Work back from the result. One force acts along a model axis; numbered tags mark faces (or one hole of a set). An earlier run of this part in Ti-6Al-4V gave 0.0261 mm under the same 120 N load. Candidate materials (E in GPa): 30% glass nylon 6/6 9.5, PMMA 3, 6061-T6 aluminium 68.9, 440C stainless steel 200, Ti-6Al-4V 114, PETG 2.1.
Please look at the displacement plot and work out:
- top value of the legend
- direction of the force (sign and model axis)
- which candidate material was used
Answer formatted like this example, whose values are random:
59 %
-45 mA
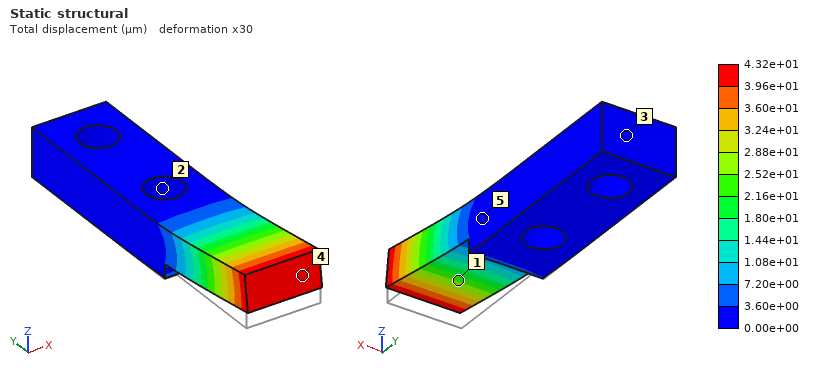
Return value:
4.32e+01 µm
+Z
6061-T6 aluminium
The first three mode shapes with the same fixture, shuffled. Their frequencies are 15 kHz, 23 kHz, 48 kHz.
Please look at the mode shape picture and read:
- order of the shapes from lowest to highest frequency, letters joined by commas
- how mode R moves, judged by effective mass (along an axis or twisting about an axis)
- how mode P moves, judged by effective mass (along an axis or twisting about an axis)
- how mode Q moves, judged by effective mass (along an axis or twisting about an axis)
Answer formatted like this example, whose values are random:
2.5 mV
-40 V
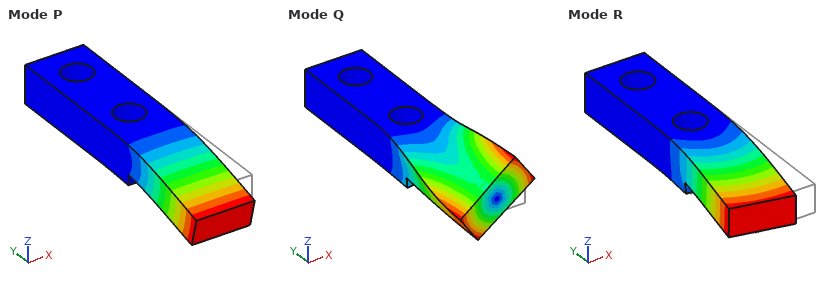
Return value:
P, R, Q
along X
along Z
twisting about Y
